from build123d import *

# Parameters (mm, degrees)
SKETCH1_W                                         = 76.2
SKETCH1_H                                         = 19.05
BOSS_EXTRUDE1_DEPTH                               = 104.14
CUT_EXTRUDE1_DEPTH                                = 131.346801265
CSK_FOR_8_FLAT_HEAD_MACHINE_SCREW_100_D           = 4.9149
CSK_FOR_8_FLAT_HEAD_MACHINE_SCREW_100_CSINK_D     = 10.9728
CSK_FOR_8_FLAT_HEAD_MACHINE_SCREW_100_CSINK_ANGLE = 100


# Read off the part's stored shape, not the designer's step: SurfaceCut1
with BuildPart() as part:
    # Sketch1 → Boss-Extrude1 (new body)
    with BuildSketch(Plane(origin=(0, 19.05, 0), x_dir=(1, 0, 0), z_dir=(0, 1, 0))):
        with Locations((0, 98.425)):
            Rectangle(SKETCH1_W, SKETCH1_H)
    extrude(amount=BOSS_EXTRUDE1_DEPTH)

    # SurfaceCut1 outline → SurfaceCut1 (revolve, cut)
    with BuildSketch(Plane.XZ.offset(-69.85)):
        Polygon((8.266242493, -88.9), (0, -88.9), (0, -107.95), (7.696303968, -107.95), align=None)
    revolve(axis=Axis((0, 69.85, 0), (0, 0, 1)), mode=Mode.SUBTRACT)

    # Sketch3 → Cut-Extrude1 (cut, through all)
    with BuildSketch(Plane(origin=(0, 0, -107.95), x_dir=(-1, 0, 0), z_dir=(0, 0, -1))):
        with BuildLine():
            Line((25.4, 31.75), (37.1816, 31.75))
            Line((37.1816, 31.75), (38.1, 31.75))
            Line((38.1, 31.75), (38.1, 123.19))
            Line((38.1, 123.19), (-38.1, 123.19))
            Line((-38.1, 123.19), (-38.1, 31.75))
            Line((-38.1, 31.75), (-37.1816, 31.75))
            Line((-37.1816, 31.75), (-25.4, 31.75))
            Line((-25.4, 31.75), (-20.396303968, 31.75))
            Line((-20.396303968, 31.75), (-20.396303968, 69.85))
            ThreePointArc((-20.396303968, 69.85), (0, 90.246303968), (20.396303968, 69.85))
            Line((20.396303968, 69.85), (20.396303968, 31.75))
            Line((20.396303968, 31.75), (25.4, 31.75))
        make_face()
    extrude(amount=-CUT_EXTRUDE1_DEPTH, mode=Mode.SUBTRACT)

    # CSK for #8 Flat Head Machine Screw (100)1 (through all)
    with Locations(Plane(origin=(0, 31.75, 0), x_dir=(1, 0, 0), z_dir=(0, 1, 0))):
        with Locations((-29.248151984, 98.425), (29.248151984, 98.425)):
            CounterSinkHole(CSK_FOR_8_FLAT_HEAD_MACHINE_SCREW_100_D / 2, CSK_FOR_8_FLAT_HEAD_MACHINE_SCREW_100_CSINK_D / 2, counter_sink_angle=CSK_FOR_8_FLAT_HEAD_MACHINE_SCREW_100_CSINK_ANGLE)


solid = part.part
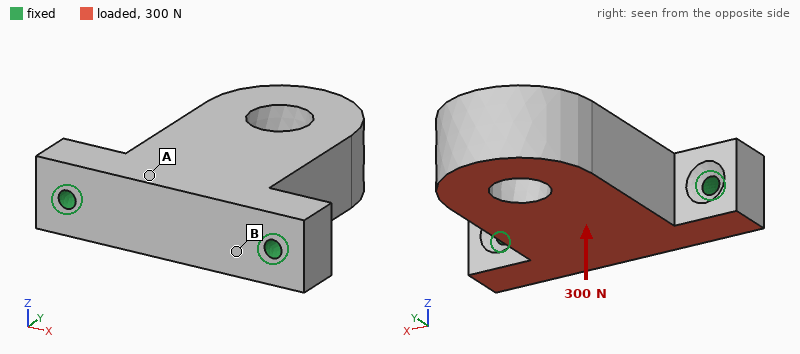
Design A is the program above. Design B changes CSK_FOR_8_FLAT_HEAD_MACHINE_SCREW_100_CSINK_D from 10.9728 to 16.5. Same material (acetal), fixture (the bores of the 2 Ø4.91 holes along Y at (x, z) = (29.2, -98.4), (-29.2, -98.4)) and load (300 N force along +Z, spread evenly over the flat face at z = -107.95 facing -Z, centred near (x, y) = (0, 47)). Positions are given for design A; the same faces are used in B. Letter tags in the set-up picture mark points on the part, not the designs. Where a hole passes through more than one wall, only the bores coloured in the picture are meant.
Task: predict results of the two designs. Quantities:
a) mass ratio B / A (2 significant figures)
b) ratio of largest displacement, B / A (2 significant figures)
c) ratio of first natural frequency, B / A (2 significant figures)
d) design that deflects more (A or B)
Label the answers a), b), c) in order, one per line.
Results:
a) 0.99
b) 1.3
c) 0.86
d) B
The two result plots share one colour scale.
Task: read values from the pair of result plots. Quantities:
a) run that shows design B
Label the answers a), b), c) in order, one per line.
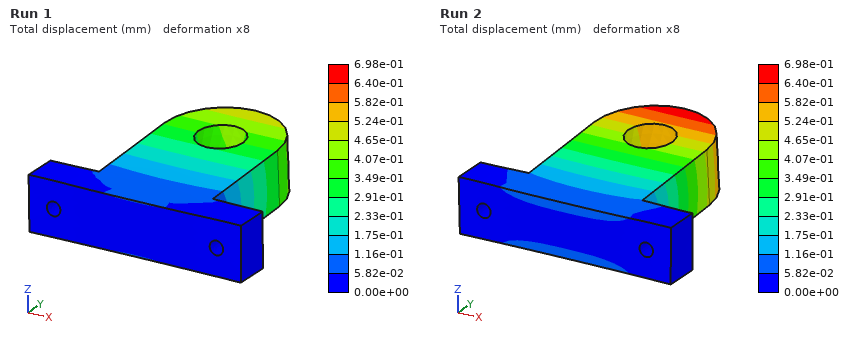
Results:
a) Run 2
